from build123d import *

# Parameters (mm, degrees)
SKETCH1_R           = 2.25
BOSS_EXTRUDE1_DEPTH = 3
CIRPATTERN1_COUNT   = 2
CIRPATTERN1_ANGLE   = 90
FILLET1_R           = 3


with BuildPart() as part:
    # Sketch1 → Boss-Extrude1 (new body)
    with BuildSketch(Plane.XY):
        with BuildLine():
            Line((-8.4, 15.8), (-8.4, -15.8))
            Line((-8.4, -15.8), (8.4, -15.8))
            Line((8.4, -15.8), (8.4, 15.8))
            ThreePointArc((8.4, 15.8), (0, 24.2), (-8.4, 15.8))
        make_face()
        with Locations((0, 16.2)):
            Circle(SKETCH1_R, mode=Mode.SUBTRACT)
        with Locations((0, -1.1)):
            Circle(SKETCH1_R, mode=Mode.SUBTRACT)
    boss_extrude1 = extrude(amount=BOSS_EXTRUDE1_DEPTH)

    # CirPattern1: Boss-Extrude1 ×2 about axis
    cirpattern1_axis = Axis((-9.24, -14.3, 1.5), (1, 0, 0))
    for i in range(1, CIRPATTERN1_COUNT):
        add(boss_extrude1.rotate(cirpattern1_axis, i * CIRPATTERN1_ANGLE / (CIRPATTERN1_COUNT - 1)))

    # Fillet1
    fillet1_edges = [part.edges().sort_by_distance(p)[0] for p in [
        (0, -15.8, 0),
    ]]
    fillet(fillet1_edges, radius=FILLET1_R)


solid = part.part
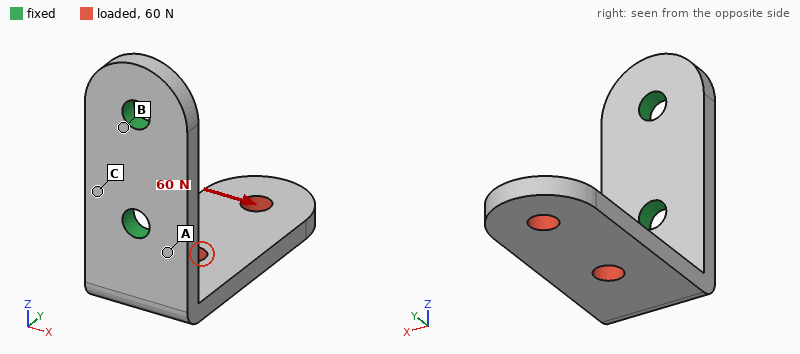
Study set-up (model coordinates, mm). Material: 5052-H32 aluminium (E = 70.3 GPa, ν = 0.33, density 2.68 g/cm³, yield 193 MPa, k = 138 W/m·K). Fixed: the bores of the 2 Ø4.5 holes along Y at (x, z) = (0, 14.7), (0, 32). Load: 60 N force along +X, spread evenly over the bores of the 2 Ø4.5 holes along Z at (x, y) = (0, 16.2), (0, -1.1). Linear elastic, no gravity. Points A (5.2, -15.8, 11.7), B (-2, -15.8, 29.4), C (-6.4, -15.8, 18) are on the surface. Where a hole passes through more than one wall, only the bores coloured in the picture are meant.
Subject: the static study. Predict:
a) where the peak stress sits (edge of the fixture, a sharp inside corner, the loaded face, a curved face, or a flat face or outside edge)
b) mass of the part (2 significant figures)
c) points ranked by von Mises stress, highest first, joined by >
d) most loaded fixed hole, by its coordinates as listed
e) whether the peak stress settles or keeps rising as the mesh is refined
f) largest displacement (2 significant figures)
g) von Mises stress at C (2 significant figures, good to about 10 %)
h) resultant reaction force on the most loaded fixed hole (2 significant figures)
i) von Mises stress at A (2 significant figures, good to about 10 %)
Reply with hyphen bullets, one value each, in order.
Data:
- edge of the fixture
- 9.3 g
- A > C > B
- (0, 14.7)
- keeps rising
- 0.14 mm
- 17 MPa
- 85 N
- 31 MPa
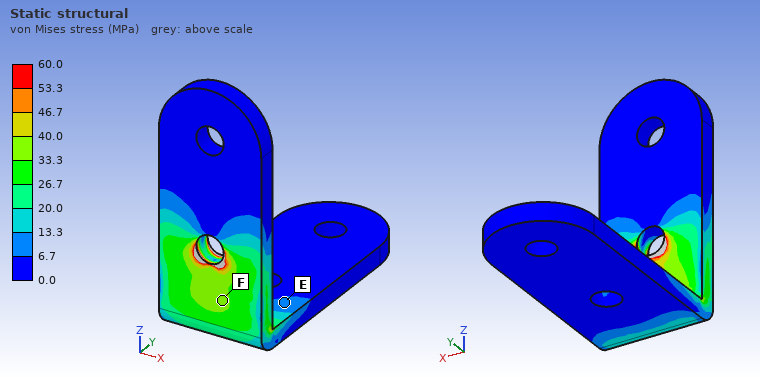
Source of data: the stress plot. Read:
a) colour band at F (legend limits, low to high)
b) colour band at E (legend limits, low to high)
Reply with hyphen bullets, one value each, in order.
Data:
- 33.3 to 40.0 MPa
- 6.7 to 13.3 MPa
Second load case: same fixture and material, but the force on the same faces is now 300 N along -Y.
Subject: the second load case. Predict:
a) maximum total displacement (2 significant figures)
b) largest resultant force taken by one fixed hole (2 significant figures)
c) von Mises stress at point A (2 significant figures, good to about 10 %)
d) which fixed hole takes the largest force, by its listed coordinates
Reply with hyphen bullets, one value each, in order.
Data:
- 0.33 mm
- 330 N
- 82 MPa
- (0, 14.7)
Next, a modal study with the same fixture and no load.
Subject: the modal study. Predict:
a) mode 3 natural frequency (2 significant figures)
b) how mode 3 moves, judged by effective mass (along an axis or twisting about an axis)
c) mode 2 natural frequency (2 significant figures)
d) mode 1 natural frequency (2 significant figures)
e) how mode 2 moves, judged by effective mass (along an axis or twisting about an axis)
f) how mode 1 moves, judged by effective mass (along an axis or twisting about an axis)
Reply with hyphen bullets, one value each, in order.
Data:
- 5600 Hz
- along Y
- 2000 Hz
- 1200 Hz
- along X
- along Z
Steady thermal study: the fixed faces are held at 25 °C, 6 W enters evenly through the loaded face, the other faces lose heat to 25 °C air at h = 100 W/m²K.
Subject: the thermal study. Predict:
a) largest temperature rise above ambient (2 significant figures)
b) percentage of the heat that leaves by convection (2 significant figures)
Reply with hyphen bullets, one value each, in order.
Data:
- 21 K
- 39 %
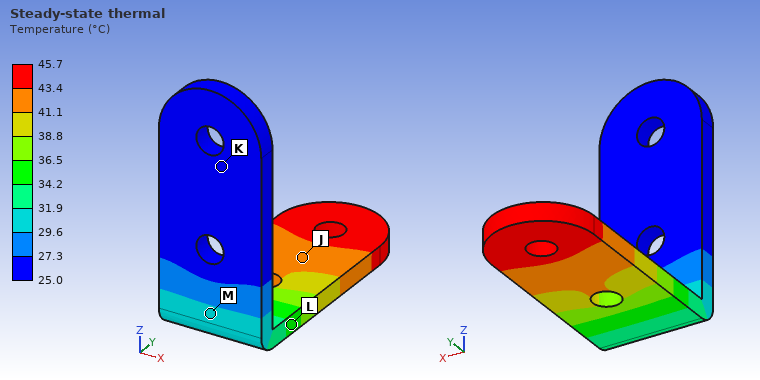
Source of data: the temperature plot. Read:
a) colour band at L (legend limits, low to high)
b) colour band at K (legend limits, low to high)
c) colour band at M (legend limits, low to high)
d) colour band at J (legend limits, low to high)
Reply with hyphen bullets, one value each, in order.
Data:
- 34.2 to 36.5 °C
- 25.0 to 27.3 °C
- 29.6 to 31.9 °C
- 41.1 to 43.4 °C
